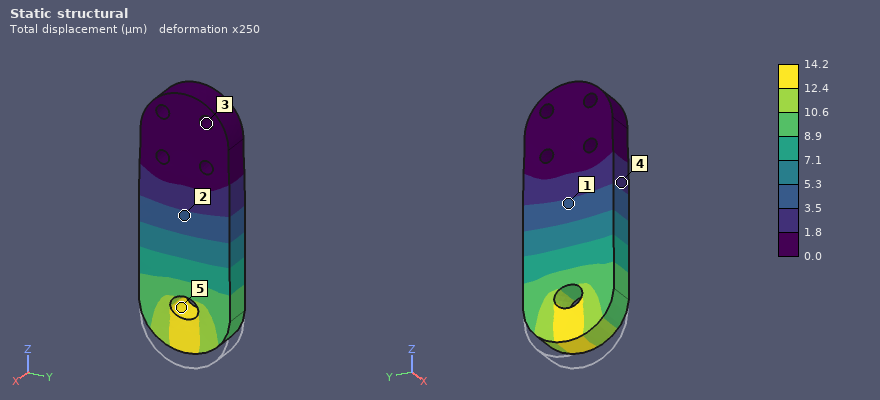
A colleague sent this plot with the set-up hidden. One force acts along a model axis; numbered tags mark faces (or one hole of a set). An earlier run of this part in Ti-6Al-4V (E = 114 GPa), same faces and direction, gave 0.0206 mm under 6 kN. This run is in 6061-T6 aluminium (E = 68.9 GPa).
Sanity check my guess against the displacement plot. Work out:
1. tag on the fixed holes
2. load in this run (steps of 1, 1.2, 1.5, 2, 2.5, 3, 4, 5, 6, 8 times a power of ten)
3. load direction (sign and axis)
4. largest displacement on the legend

3
2.5 kN
+Z
14.2 µm
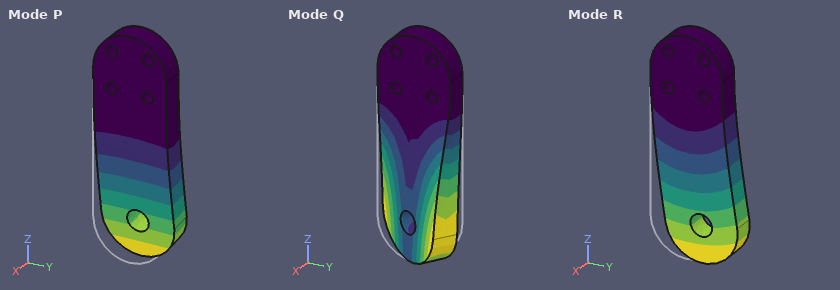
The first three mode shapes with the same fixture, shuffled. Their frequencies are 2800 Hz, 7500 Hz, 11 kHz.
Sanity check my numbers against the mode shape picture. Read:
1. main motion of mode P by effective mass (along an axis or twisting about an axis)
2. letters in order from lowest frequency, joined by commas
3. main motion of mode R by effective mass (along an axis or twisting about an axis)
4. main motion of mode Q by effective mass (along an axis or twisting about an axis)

along X
P, R, Q
along Y
twisting about Z
